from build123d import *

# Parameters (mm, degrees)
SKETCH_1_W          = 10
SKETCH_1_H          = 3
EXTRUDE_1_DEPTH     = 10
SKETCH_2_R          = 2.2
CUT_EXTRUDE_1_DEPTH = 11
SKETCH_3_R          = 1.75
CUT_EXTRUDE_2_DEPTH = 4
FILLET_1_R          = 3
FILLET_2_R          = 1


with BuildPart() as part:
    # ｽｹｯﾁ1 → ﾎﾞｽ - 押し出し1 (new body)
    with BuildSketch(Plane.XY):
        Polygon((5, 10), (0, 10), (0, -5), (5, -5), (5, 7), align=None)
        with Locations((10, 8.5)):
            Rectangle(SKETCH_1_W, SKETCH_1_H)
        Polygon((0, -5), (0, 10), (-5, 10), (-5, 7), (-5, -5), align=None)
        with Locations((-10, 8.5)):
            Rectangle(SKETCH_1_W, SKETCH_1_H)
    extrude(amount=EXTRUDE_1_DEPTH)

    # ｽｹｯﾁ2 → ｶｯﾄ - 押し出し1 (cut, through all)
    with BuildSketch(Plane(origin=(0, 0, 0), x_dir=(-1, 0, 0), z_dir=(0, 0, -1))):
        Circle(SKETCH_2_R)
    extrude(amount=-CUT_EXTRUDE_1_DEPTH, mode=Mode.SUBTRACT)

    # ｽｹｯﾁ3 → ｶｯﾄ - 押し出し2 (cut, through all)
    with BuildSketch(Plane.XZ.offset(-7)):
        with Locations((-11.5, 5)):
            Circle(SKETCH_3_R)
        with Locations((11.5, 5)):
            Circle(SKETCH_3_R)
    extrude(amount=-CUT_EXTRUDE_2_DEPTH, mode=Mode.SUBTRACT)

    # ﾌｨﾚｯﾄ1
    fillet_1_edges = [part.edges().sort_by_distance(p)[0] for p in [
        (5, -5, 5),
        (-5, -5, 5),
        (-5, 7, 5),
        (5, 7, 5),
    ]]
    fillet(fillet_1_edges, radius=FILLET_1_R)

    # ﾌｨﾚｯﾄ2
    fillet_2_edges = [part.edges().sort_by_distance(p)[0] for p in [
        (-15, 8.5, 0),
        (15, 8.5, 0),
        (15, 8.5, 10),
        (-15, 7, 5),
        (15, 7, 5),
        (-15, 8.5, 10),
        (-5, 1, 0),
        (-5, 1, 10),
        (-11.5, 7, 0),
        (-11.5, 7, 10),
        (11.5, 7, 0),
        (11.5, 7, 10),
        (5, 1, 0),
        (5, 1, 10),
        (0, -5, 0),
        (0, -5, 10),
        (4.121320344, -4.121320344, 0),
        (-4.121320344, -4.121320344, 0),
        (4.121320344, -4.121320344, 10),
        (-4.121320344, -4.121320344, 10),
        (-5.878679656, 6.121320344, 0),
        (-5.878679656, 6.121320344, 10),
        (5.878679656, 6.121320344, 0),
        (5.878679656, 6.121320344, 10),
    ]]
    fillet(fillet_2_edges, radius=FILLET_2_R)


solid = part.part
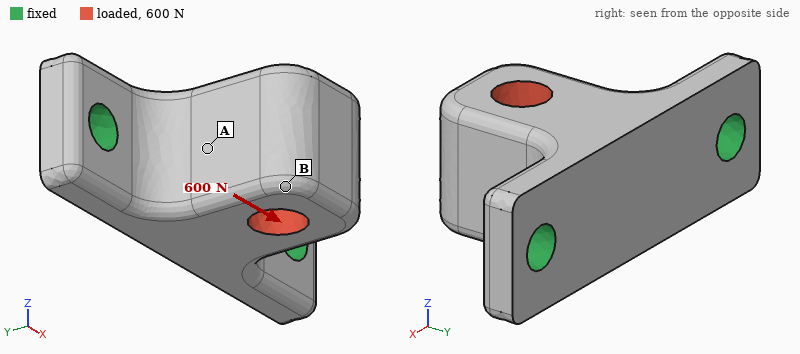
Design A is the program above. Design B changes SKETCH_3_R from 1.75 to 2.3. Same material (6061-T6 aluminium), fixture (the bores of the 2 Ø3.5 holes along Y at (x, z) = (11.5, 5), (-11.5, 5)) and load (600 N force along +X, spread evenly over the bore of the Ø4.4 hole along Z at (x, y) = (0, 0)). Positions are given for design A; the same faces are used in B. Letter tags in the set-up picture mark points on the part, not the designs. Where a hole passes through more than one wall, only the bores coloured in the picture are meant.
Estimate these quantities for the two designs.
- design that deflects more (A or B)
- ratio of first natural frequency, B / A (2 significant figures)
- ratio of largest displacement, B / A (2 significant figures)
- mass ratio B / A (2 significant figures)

A
1.1
0.89
0.98
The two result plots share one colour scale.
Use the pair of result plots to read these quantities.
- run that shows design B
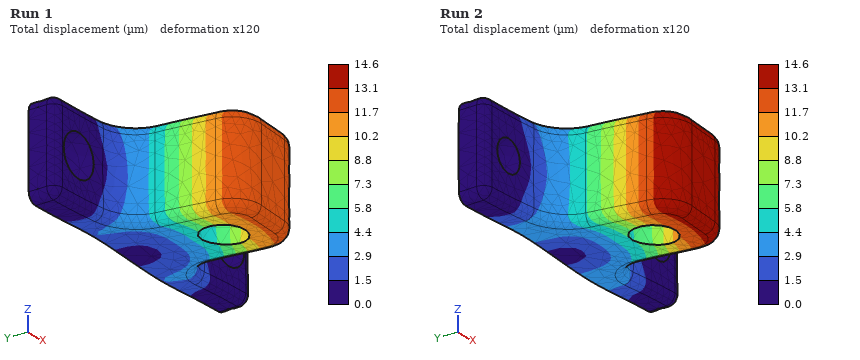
Run 1
